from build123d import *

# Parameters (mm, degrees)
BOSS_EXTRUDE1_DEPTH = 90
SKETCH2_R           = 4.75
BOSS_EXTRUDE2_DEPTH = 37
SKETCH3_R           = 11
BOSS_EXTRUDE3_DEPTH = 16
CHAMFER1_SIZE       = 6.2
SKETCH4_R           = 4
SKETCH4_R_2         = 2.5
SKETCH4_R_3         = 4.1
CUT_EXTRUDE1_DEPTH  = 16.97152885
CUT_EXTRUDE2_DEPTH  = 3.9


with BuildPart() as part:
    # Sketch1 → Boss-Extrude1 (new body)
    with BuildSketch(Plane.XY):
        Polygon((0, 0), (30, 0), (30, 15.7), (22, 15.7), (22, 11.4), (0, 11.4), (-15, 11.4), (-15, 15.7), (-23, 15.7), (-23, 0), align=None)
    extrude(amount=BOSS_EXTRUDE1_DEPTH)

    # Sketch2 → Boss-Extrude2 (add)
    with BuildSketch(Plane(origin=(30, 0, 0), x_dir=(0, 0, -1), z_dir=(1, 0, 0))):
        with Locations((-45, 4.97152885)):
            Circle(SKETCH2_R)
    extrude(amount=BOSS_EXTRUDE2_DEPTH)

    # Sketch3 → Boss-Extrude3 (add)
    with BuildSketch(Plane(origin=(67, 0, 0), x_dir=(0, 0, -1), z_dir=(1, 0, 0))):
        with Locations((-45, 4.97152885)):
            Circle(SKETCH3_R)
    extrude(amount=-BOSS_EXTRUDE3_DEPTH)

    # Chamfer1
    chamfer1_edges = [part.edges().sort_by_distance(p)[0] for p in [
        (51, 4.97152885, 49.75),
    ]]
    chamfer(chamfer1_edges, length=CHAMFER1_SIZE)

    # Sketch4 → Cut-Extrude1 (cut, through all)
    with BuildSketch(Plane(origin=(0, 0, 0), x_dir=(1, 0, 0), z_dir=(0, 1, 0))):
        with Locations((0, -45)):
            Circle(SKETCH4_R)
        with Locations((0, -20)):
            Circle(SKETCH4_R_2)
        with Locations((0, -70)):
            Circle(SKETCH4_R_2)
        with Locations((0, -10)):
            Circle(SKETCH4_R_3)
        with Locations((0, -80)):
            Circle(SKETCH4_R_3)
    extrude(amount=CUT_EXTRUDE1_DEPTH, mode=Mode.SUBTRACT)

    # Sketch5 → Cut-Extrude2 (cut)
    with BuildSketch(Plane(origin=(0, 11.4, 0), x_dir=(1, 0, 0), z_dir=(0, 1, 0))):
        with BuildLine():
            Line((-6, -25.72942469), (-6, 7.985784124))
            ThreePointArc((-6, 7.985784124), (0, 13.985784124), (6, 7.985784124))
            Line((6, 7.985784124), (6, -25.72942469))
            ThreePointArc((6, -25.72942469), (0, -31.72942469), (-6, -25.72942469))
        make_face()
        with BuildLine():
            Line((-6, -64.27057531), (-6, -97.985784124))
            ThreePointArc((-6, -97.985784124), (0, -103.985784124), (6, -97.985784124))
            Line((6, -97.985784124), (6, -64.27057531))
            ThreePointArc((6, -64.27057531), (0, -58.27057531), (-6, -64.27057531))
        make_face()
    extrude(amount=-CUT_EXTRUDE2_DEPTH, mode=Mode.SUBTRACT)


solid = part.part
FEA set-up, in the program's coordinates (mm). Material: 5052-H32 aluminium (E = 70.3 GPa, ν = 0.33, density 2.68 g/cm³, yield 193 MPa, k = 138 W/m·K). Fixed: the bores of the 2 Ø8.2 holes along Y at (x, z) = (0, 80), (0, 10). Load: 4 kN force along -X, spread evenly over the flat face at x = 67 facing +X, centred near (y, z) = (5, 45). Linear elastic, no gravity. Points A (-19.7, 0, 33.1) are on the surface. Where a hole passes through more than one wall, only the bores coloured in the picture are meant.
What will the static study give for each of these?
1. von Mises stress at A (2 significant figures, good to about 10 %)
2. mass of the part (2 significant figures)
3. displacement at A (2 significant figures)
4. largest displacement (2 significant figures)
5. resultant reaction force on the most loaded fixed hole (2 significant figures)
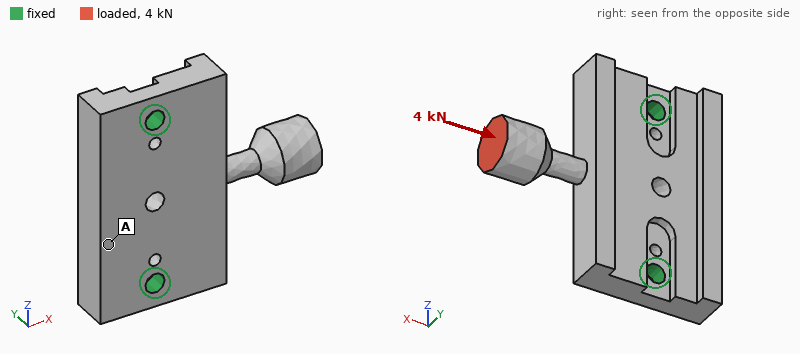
7.0 MPa
170 g
5.6 µm
31 µm
2.1 kN
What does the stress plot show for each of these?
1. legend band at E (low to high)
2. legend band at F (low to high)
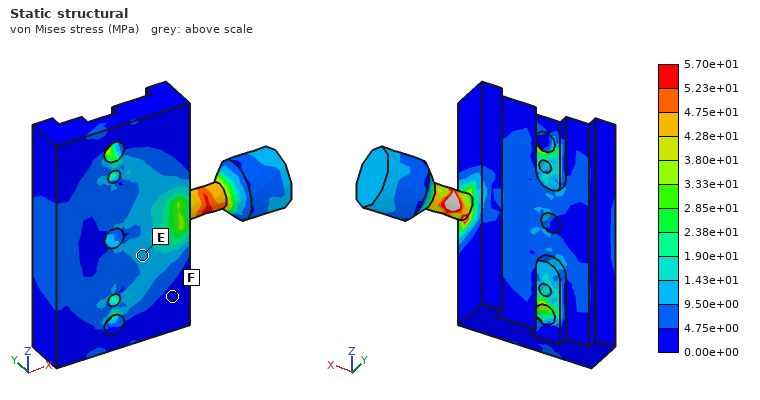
9.50e+00 to 1.43e+01 MPa
0.00e+00 to 4.75e+00 MPa
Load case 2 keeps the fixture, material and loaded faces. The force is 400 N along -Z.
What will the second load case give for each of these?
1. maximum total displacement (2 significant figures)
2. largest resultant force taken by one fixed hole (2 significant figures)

0.26 mm
420 N
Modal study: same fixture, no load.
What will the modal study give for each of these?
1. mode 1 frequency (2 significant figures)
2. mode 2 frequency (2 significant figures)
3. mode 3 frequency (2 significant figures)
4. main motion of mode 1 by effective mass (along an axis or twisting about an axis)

1500 Hz
1900 Hz
4900 Hz
along Y
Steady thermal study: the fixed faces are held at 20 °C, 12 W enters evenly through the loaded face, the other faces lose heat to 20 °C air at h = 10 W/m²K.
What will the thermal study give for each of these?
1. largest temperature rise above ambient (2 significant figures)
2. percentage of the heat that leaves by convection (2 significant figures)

33 K
7.1 %
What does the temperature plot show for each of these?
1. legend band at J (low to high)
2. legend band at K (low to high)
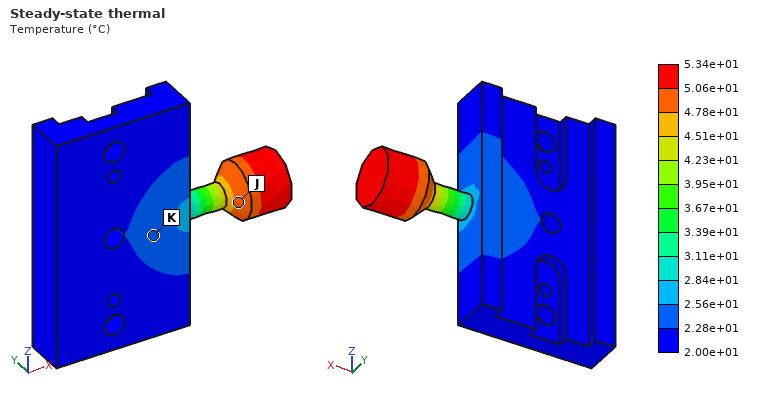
4.78e+01 to 5.06e+01 °C
2.28e+01 to 2.56e+01 °C
